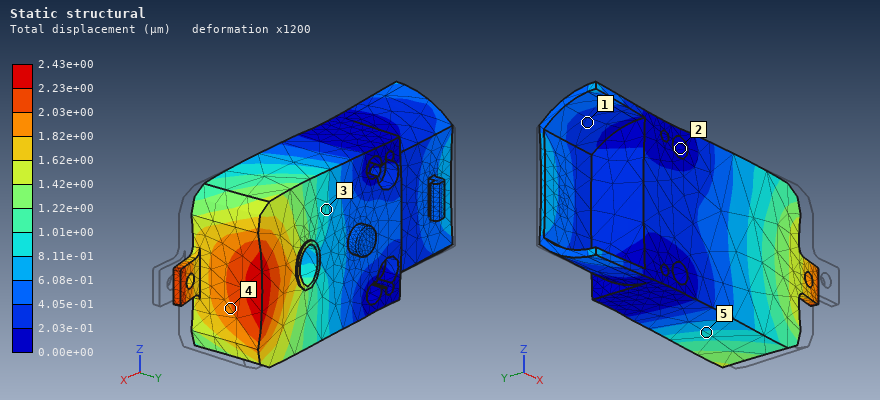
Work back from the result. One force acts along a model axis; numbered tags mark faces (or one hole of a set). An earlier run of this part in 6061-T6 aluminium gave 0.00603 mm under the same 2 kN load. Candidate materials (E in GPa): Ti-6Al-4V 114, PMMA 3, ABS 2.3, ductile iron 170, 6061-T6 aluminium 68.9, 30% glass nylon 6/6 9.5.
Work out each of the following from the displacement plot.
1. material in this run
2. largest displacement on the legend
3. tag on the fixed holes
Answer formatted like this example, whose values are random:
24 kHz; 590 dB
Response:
ductile iron; 2.43e+00 µm; 2
